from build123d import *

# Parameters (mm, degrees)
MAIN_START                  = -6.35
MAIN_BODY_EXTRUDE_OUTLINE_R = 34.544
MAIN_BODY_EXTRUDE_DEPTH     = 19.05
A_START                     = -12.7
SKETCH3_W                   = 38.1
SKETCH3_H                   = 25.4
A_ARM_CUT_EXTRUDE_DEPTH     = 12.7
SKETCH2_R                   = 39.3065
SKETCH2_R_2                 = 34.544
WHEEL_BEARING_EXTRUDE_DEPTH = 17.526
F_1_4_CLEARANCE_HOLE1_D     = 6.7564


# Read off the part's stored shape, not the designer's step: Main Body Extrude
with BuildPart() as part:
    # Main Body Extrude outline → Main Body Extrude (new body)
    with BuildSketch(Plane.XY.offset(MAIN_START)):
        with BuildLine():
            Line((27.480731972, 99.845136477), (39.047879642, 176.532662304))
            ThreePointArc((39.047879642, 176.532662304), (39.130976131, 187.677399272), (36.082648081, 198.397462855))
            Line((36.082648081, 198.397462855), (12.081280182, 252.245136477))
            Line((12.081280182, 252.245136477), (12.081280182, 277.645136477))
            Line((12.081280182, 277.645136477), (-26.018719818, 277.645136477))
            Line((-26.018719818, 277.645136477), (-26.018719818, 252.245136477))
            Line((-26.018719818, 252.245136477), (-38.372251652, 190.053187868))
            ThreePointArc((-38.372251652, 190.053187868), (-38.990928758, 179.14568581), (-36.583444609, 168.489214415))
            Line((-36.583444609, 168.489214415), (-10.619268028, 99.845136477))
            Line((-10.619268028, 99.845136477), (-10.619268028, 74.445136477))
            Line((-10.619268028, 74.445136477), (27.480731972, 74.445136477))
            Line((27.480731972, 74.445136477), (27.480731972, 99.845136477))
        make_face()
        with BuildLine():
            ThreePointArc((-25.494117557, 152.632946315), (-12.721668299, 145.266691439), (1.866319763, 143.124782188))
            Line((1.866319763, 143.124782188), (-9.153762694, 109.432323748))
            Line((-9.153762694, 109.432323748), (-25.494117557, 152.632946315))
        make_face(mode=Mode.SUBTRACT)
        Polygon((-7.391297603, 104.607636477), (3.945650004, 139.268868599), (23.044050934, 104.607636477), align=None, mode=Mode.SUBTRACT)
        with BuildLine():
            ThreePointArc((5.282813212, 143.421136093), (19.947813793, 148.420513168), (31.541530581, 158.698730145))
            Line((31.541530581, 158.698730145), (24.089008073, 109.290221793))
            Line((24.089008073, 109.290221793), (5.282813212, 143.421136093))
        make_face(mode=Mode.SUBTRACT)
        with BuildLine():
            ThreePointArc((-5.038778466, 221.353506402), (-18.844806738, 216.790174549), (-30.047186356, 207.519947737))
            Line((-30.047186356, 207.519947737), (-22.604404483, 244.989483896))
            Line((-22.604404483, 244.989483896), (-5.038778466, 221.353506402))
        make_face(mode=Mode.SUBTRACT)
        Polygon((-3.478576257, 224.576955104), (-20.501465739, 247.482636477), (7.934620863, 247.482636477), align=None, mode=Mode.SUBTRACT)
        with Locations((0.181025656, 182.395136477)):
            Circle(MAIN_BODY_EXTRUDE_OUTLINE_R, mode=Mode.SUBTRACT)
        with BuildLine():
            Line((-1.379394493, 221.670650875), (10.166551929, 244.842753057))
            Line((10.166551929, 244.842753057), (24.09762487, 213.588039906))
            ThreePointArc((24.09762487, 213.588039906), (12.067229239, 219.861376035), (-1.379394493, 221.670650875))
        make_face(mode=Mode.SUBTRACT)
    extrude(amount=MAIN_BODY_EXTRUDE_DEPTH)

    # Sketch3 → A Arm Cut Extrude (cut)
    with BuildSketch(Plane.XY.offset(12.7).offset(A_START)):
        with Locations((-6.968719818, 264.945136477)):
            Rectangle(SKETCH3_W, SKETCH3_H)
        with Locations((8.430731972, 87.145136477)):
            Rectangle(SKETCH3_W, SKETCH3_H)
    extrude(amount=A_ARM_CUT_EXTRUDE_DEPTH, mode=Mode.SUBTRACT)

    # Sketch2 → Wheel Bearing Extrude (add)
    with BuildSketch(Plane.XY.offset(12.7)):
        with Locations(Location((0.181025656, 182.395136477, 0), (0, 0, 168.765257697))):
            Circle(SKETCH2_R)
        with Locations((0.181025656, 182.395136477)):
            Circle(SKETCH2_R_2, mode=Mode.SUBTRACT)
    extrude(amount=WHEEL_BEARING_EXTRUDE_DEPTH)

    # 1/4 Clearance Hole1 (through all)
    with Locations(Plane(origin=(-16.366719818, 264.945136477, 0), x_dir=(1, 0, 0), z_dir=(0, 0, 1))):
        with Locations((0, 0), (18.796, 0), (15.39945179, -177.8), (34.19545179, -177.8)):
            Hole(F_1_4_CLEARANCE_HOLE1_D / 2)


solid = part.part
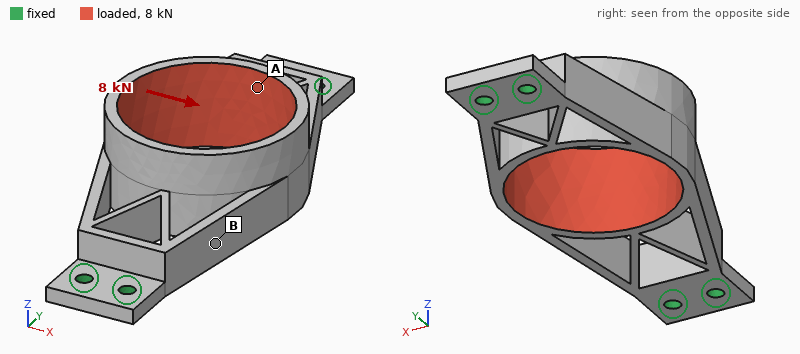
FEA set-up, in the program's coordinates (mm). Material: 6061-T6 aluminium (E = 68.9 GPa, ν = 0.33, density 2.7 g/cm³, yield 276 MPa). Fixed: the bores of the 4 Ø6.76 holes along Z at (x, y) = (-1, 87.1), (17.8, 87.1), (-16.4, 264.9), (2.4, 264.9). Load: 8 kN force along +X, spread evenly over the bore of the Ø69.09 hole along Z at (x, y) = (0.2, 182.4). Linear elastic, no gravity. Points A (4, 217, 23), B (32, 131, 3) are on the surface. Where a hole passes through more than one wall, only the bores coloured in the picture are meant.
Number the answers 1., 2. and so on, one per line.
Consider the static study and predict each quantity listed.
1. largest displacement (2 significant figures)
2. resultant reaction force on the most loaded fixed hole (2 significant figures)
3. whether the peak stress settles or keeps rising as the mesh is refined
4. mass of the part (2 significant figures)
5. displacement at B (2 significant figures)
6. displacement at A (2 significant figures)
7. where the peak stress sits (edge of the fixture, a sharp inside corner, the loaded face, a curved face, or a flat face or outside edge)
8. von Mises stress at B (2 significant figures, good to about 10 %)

1. 0.46 mm
2. 5.2 kN
3. keeps rising
4. 230 g
5. 0.19 mm
6. 0.24 mm
7. edge of the fixture
8. 36 MPa
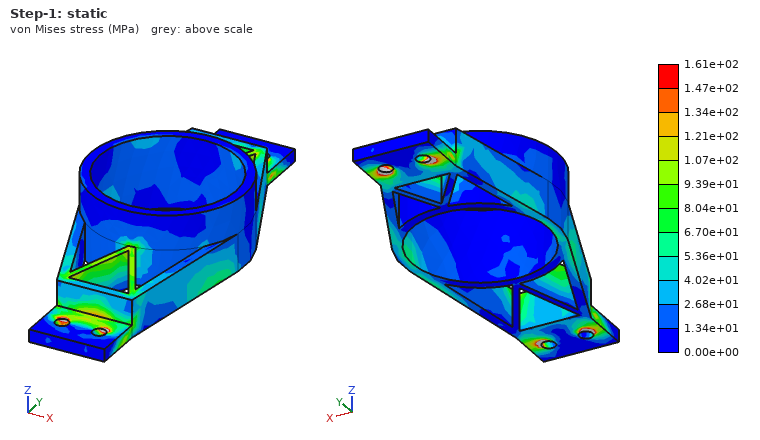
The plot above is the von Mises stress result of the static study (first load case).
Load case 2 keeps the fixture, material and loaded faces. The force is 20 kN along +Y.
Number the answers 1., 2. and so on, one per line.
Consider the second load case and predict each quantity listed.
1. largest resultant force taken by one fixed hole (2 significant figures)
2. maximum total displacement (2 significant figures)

1. 6.1 kN
2. 0.17 mm
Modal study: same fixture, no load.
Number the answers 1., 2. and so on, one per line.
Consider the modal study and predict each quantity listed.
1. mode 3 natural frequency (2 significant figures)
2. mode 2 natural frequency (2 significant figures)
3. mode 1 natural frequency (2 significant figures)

1. 2800 Hz
2. 1500 Hz
3. 1500 Hz
